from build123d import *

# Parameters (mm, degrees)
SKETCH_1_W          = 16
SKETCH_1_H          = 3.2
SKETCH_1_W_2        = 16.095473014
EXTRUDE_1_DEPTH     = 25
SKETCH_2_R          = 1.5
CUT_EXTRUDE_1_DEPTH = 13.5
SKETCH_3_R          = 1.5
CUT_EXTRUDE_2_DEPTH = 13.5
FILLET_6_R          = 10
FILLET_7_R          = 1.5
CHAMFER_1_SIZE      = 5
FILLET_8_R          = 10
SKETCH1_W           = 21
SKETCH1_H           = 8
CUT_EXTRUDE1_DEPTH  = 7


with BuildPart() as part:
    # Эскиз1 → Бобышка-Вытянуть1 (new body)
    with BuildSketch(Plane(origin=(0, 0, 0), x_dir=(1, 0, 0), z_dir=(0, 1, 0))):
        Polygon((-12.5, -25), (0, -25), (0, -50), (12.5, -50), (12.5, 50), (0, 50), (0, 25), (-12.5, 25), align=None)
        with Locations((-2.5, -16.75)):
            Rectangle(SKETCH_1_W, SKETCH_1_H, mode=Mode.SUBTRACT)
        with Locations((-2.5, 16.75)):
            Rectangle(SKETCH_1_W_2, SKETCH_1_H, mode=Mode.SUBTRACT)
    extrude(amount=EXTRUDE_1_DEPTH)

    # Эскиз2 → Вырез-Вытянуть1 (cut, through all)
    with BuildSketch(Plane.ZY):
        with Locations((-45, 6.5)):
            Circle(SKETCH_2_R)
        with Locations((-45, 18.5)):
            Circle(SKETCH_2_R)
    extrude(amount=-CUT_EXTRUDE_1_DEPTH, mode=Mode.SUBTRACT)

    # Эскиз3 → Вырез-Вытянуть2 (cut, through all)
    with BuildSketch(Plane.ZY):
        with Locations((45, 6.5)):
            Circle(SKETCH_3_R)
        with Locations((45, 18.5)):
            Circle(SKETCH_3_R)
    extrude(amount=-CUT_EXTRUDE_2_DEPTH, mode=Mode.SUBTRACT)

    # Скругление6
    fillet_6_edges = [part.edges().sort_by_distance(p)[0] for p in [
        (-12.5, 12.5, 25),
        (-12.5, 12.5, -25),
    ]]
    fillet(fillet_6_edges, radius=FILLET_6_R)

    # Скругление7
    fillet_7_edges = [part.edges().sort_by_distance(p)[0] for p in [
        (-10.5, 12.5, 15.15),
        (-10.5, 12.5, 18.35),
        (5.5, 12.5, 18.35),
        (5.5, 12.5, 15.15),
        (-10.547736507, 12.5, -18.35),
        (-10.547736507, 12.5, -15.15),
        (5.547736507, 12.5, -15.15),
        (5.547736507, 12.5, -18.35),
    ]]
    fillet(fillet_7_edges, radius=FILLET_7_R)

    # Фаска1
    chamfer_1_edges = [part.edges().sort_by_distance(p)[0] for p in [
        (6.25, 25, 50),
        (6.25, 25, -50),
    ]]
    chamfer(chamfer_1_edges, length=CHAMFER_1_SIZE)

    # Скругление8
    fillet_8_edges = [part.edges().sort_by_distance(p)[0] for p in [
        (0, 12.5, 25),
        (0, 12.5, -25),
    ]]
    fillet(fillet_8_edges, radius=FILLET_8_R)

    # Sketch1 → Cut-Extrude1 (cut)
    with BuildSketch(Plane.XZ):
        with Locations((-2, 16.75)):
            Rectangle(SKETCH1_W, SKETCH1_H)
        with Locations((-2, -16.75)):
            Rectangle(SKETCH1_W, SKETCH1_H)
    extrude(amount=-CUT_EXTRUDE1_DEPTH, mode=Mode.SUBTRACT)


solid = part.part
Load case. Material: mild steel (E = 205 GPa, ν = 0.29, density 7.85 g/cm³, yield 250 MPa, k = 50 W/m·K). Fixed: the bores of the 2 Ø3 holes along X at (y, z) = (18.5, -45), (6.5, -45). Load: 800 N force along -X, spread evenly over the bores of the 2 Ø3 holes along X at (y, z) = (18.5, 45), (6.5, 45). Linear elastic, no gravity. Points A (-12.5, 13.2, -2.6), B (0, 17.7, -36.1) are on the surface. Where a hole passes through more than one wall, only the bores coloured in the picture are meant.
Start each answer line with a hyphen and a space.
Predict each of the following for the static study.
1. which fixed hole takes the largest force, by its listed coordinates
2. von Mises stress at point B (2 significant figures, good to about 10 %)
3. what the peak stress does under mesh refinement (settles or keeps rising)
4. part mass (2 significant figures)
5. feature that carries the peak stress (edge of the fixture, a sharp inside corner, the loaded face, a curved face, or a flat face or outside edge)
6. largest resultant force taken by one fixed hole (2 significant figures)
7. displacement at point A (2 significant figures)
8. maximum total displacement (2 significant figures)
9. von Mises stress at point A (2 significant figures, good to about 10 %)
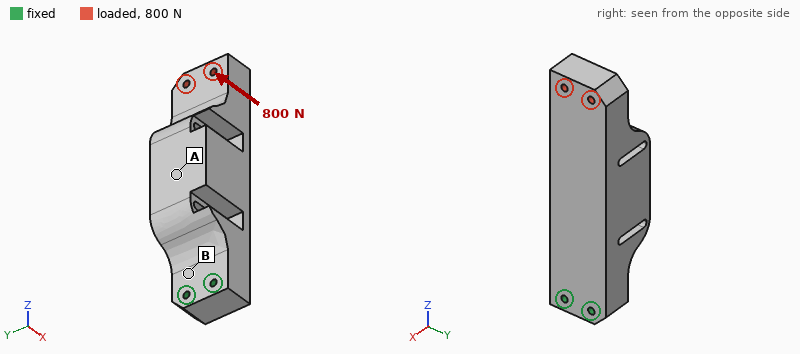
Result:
- (6.5, -45)
- 110 MPa
- keeps rising
- 330 g
- edge of the fixture
- 450 N
- 0.080 mm
- 0.21 mm
- 23 MPa
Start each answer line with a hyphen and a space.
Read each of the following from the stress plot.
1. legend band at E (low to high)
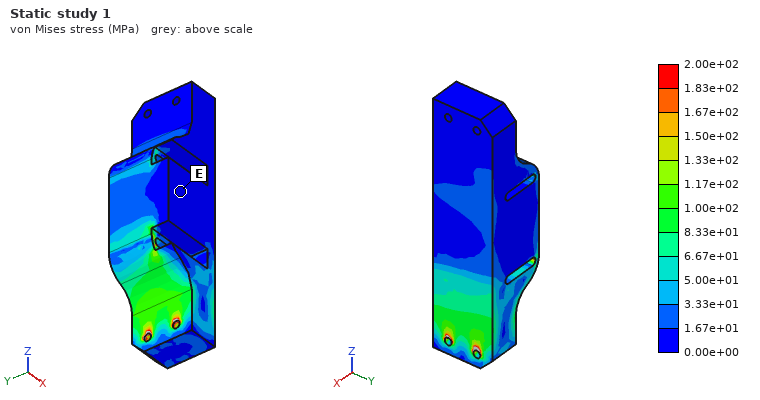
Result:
- 0.00e+00 to 1.67e+01 MPa
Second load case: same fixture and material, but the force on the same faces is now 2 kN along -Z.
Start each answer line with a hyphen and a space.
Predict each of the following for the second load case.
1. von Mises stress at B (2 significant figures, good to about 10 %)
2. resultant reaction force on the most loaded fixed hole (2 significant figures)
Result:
- 7.8 MPa
- 1.0 kN
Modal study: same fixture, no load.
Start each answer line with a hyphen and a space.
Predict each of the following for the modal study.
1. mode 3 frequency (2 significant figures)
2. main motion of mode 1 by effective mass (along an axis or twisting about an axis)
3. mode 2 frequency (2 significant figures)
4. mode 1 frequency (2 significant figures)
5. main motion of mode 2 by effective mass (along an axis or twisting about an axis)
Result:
- 5300 Hz
- along X
- 1700 Hz
- 1100 Hz
- along Y
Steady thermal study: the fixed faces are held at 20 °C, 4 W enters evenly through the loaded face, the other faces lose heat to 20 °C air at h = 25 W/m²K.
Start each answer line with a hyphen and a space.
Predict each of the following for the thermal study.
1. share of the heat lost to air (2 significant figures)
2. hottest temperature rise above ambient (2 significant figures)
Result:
- 48 %
- 16 K
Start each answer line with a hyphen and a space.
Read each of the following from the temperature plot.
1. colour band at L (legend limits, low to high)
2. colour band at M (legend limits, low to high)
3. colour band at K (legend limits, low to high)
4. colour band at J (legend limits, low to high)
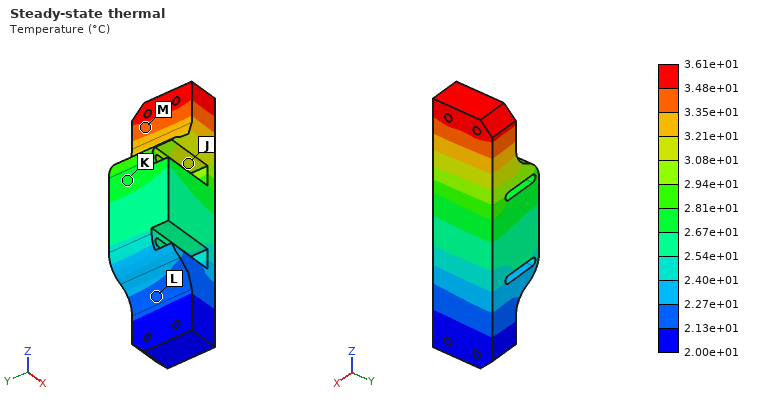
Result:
- 2.13e+01 to 2.27e+01 °C
- 3.35e+01 to 3.48e+01 °C
- 2.67e+01 to 2.81e+01 °C
- 3.08e+01 to 3.21e+01 °C
